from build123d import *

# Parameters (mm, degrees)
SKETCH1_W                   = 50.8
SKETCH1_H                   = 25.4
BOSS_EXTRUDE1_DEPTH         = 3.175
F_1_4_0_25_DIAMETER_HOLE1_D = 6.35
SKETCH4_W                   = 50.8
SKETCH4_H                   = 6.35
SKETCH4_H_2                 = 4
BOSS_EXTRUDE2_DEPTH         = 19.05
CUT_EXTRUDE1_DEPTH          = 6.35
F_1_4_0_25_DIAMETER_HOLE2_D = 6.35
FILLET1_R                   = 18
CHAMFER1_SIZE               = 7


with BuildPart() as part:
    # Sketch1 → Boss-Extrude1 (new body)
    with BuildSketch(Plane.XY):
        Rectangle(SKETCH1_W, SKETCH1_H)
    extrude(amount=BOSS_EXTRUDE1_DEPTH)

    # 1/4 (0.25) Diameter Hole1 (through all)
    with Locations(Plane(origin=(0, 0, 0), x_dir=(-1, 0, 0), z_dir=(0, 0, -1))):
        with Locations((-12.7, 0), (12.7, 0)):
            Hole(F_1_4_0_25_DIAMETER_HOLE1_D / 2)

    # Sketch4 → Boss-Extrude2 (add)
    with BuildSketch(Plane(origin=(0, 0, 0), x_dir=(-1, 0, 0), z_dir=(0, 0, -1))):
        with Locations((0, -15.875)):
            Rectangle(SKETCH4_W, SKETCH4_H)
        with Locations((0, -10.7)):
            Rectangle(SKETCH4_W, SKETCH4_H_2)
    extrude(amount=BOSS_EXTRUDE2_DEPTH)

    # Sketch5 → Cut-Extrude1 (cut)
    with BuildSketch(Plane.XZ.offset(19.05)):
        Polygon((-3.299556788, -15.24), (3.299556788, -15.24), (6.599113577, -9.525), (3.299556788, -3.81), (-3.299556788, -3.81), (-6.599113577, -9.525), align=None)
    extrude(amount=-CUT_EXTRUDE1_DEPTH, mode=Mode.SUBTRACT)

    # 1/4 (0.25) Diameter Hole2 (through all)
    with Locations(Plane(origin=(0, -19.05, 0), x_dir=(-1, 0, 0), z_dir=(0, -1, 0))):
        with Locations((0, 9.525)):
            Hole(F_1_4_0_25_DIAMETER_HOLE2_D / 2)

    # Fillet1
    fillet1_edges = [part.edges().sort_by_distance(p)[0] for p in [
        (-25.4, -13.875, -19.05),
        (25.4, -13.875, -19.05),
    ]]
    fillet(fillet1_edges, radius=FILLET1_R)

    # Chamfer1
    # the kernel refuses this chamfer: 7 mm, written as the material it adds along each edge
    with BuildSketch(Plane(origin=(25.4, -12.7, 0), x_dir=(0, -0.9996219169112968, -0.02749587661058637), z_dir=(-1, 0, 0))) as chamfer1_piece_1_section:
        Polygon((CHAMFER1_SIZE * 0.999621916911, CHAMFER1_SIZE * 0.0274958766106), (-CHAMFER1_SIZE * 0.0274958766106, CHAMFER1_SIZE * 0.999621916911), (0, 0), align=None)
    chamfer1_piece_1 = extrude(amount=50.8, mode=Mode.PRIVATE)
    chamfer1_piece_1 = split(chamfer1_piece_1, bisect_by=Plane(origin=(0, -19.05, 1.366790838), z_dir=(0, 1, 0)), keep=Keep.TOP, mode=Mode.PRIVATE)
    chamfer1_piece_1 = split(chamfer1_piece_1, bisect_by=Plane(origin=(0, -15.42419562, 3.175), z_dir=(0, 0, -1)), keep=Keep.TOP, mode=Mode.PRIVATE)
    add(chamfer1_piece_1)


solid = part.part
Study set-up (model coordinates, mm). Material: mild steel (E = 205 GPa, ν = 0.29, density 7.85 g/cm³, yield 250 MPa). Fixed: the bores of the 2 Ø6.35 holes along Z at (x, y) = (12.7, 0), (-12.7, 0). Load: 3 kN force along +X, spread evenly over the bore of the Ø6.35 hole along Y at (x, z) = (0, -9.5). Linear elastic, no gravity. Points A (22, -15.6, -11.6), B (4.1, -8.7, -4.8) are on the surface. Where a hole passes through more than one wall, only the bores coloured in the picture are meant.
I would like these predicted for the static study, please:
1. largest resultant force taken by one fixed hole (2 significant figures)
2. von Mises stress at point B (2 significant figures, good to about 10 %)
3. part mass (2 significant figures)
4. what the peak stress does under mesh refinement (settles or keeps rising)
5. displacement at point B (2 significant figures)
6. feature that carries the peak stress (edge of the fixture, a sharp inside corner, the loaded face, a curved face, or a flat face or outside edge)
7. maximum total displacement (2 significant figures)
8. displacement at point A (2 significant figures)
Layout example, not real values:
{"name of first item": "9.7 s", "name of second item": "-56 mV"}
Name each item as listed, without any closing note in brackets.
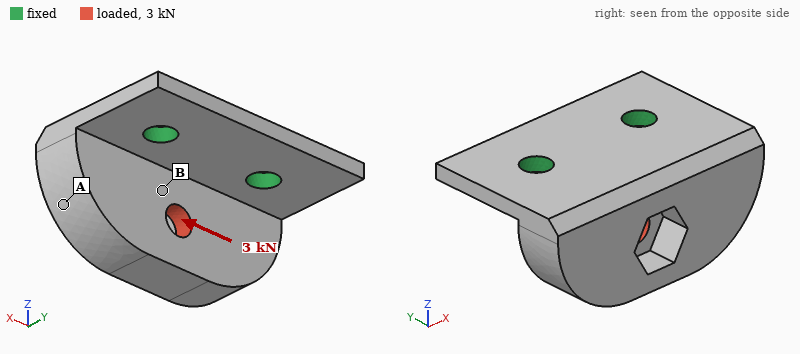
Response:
{"largest resultant force taken by one fixed hole": "2.1 kN", "von Mises stress at point B": "49 MPa", "part mass": "98 g", "what the peak stress does under mesh refinement": "keeps rising", "displacement at point B": "9.3 µm", "feature that carries the peak stress": "edge of the fixture", "maximum total displacement": "24 µm", "displacement at point A": "23 µm"}
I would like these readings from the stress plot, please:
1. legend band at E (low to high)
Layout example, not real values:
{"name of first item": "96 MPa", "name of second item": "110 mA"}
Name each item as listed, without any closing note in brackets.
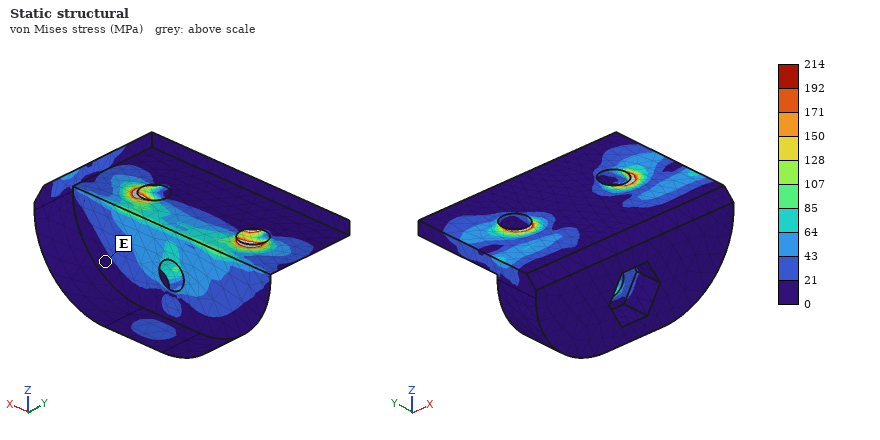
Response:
{"legend band at E": "0 to 21 MPa"}
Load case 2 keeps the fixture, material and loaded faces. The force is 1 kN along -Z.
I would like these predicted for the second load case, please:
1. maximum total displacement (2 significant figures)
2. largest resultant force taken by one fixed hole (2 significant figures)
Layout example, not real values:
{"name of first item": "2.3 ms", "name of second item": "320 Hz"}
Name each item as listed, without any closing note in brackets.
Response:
{"maximum total displacement": "40 µm", "largest resultant force taken by one fixed hole": "500 N"}
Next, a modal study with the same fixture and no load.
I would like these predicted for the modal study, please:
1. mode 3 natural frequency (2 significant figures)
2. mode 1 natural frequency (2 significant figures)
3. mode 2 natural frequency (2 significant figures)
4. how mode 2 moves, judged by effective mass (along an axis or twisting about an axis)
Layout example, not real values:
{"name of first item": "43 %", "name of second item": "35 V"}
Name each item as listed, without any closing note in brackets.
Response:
{"mode 3 natural frequency": "12 kHz", "mode 1 natural frequency": "2400 Hz", "mode 2 natural frequency": "6700 Hz", "how mode 2 moves, judged by effective mass": "along X"}
